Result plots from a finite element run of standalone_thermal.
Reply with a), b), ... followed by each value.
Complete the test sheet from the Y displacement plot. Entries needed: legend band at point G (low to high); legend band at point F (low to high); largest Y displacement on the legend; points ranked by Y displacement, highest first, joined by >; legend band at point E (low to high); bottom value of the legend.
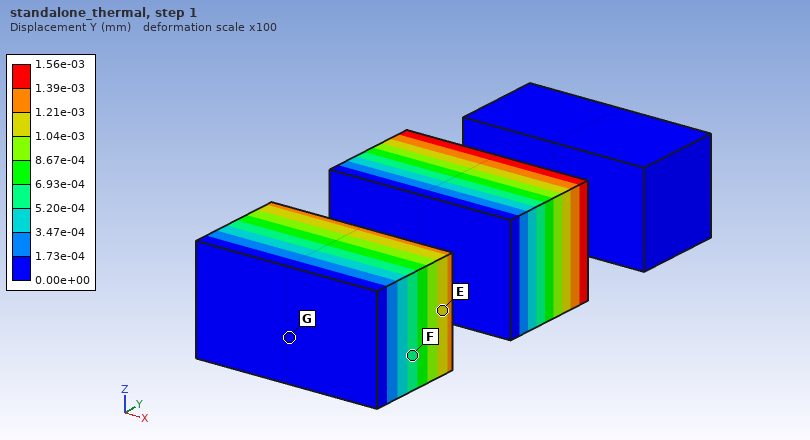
a) 0.00e+00 to 1.73e-04 mm
b) 5.20e-04 to 6.93e-04 mm
c) 1.56e-03 mm
d) E > F > G
e) 1.04e-03 to 1.21e-03 mm
f) 0.00e+00 mm
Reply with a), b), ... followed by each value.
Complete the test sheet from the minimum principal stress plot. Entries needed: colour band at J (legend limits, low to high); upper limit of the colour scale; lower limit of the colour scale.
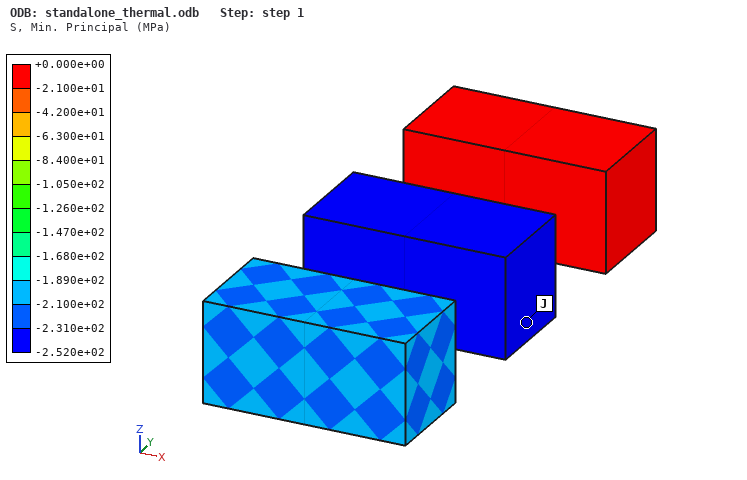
a) -2.520e+02 to -2.310e+02 MPa
b) +0.000e+00 MPa
c) -2.520e+02 MPa
